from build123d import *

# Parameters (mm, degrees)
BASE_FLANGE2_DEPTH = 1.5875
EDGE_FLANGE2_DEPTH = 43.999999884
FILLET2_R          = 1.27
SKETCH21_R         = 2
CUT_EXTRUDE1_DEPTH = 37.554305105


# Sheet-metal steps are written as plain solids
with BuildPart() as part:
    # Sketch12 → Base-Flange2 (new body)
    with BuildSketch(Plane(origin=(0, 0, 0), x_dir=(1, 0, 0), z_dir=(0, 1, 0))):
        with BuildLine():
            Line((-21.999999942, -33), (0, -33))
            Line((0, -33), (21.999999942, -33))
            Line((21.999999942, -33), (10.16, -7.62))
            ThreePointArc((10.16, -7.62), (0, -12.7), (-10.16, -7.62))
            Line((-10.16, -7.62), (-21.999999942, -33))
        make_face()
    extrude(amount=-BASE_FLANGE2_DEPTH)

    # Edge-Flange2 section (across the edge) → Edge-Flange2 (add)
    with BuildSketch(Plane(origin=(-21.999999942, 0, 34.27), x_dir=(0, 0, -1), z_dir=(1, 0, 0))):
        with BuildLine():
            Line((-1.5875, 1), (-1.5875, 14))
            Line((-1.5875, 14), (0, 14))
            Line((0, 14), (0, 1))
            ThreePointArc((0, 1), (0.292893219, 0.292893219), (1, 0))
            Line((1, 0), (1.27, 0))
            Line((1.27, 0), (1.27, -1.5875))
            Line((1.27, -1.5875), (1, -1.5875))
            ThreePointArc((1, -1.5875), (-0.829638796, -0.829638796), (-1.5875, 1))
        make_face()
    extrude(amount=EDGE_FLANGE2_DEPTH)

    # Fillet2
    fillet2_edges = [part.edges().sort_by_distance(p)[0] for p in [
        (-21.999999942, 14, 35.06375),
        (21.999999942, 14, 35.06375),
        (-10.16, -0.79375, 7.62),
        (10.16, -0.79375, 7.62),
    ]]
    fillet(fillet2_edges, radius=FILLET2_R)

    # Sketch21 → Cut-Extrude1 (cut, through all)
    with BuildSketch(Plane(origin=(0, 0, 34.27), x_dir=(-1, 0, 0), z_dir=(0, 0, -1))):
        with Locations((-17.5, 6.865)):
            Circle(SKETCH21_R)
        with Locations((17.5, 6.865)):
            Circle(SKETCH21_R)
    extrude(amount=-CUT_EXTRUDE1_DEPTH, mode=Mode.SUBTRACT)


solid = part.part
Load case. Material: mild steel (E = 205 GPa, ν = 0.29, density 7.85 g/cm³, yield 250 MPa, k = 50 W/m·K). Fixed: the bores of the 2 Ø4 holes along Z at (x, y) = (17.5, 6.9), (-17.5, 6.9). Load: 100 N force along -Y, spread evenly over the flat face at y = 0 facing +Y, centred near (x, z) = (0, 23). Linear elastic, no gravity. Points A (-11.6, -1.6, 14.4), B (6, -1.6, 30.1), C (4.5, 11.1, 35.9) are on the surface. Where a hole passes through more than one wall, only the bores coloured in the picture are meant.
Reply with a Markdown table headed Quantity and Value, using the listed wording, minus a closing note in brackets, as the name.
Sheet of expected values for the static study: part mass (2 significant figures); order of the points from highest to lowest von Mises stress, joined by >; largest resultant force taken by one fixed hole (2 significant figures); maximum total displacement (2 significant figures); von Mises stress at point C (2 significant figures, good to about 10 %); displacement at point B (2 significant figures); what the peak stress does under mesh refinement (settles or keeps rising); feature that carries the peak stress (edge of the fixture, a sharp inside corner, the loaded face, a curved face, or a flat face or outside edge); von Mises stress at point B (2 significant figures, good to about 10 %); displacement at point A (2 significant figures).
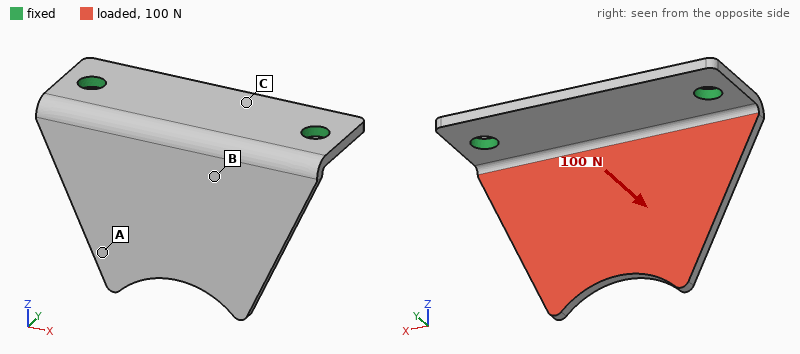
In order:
| Quantity | Value |
|---|---|
| part mass | 18 g |
| order of the points from highest to lowest von Mises stress, joined by > | B > C > A |
| largest resultant force taken by one fixed hole | 51 N |
| maximum total displacement | 0.14 mm |
| von Mises stress at point C | 21 MPa |
| displacement at point B | 0.024 mm |
| what the peak stress does under mesh refinement | keeps rising |
| feature that carries the peak stress | edge of the fixture |
| von Mises stress at point B | 38 MPa |
| displacement at point A | 0.11 mm |
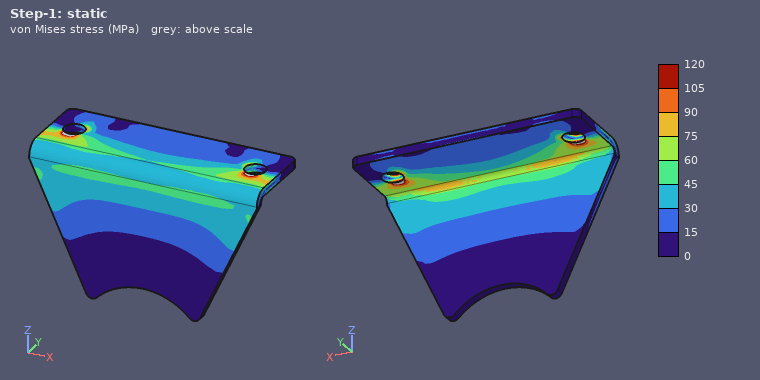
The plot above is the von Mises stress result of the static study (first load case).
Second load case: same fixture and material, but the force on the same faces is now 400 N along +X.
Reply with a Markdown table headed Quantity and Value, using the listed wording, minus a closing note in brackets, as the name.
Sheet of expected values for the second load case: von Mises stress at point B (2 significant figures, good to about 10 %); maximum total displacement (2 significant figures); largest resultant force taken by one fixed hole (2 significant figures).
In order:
| Quantity | Value |
|---|---|
| von Mises stress at point B | 15 MPa |
| maximum total displacement | 31 µm |
| largest resultant force taken by one fixed hole | 250 N |
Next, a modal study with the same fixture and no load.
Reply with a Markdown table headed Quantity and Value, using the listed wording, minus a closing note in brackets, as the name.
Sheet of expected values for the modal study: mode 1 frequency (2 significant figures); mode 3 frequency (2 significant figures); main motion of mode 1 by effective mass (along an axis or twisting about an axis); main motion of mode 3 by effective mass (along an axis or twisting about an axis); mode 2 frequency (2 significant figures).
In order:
| Quantity | Value |
|---|---|
| mode 1 frequency | 1800 Hz |
| mode 3 frequency | 7400 Hz |
| main motion of mode 1 by effective mass | along Y |
| main motion of mode 3 by effective mass | along Z |
| mode 2 frequency | 4600 Hz |
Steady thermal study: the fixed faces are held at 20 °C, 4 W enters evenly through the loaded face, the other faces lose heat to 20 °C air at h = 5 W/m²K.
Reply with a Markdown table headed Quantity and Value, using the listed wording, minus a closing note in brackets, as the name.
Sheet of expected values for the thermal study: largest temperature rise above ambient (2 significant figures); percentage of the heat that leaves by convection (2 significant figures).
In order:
| Quantity | Value |
|---|---|
| largest temperature rise above ambient | 28 K |
| percentage of the heat that leaves by convection | 3.8 % |
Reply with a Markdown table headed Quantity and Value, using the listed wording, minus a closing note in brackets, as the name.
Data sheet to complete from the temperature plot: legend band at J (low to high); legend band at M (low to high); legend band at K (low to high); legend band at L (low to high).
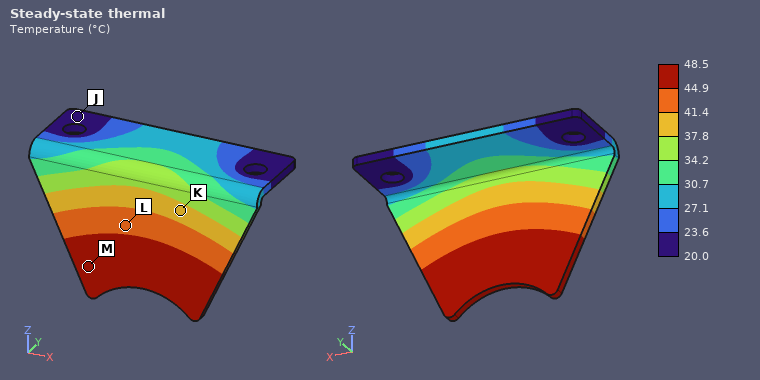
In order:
| Quantity | Value |
|---|---|
| legend band at J | 20.0 to 23.6 °C |
| legend band at M | 44.9 to 48.5 °C |
| legend band at K | 37.8 to 41.4 °C |
| legend band at L | 41.4 to 44.9 °C |
